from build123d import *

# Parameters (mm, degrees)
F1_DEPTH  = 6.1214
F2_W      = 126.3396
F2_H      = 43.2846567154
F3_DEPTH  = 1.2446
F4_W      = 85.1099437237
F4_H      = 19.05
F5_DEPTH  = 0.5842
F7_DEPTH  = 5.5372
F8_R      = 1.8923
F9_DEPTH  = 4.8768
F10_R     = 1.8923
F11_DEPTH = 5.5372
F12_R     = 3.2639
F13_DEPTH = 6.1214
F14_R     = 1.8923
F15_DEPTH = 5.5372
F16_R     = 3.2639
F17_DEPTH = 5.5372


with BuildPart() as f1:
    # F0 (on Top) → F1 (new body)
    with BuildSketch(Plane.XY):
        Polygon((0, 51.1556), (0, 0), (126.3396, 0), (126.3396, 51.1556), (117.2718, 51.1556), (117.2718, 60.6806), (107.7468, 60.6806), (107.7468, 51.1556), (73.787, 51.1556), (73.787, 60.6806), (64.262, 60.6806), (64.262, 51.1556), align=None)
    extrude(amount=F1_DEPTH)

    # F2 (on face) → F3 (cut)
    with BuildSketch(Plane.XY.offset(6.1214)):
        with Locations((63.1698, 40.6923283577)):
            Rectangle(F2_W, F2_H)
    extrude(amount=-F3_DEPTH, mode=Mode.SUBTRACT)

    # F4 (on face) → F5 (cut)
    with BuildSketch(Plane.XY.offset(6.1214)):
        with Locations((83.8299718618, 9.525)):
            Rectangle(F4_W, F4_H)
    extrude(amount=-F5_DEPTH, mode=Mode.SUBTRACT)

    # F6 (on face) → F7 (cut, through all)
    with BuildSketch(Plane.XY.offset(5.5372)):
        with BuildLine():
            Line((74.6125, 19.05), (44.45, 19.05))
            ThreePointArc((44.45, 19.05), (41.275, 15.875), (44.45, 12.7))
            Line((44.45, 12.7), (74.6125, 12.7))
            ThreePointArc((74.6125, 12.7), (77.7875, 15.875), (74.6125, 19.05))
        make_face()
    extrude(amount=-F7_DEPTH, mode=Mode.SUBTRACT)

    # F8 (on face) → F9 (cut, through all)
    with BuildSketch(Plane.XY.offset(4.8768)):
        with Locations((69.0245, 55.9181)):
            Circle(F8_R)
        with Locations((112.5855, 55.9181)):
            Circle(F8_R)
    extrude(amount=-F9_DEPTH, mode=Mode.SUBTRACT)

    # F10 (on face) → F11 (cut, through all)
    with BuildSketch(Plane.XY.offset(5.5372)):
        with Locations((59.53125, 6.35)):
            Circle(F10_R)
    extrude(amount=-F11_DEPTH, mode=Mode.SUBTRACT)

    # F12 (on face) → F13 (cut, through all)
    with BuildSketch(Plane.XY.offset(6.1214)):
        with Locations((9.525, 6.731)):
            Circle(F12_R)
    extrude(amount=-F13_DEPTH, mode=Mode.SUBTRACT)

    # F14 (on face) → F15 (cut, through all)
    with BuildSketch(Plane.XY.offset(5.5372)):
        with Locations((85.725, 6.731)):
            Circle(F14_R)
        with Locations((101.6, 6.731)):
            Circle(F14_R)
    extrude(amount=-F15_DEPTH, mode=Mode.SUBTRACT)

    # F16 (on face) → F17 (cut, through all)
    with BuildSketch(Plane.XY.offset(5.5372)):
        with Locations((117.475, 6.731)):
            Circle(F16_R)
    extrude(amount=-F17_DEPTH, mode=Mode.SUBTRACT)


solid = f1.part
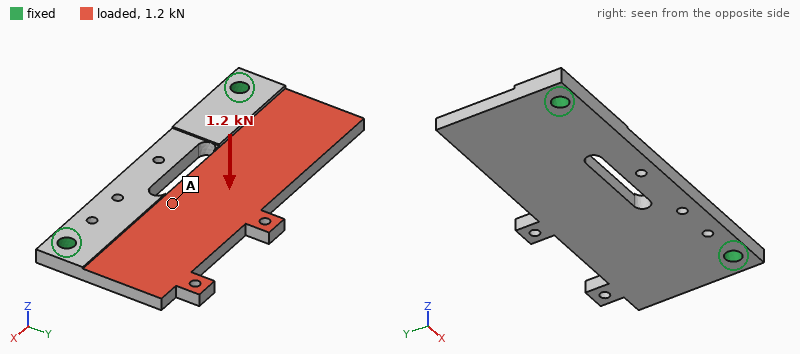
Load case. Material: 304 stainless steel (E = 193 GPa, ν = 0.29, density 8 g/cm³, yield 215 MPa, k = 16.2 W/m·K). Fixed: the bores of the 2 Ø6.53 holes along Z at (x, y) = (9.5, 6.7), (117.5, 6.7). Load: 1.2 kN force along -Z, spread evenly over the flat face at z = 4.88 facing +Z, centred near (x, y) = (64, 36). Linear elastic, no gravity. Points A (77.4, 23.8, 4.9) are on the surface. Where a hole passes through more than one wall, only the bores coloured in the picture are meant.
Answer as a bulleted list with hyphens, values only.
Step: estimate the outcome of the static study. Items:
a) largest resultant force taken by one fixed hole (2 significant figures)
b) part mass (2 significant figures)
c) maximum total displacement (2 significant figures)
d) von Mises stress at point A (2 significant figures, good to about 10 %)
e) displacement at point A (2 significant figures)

- 610 N
- 260 g
- 0.21 mm
- 24 MPa
- 0.073 mm
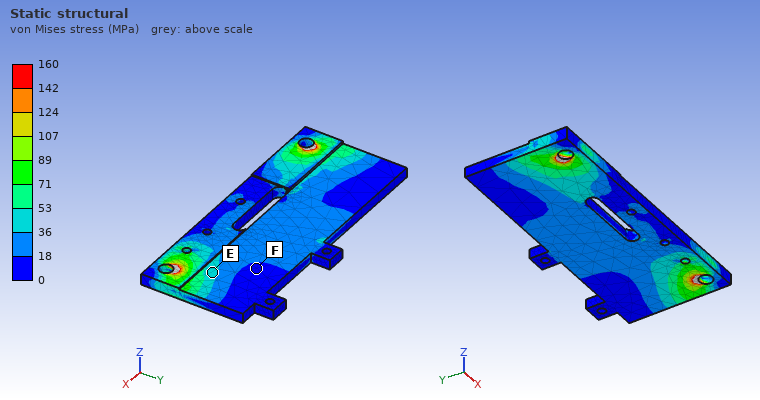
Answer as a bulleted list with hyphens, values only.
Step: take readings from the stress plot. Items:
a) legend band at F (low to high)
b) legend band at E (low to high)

- 0 to 18 MPa
- 36 to 53 MPa
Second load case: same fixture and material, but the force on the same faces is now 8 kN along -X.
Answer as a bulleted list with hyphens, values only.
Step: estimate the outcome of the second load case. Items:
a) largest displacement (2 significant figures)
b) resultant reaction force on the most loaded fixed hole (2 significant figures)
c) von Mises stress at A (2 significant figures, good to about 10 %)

- 37 µm
- 4.6 kN
- 32 MPa
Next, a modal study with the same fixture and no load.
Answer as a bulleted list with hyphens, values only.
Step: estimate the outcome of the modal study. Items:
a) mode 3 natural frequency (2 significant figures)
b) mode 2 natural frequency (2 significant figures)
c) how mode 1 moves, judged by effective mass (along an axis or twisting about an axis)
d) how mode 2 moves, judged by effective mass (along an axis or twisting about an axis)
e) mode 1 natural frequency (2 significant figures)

- 2800 Hz
- 2500 Hz
- along Z
- twisting about Y
- 1300 Hz
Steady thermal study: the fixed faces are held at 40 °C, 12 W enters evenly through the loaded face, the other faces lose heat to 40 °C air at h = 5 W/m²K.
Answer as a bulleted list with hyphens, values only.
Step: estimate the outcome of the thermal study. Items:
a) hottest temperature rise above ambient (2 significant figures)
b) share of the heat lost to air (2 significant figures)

- 64 K
- 17 %
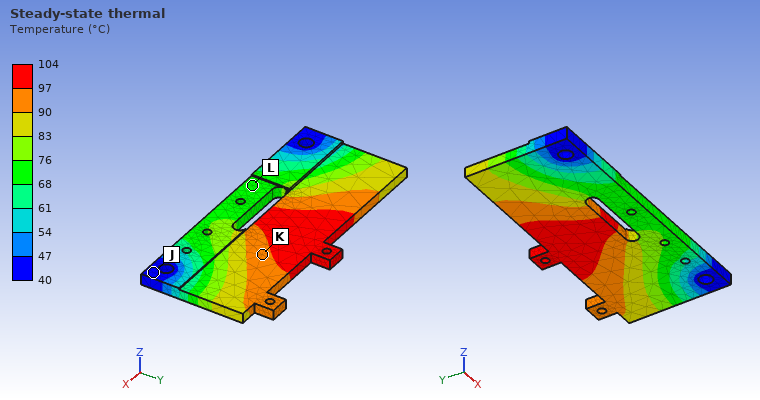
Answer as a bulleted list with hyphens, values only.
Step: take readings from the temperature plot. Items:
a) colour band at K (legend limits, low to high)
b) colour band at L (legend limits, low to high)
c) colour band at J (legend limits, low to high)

- 90 to 97 °C
- 68 to 76 °C
- 40 to 47 °C
